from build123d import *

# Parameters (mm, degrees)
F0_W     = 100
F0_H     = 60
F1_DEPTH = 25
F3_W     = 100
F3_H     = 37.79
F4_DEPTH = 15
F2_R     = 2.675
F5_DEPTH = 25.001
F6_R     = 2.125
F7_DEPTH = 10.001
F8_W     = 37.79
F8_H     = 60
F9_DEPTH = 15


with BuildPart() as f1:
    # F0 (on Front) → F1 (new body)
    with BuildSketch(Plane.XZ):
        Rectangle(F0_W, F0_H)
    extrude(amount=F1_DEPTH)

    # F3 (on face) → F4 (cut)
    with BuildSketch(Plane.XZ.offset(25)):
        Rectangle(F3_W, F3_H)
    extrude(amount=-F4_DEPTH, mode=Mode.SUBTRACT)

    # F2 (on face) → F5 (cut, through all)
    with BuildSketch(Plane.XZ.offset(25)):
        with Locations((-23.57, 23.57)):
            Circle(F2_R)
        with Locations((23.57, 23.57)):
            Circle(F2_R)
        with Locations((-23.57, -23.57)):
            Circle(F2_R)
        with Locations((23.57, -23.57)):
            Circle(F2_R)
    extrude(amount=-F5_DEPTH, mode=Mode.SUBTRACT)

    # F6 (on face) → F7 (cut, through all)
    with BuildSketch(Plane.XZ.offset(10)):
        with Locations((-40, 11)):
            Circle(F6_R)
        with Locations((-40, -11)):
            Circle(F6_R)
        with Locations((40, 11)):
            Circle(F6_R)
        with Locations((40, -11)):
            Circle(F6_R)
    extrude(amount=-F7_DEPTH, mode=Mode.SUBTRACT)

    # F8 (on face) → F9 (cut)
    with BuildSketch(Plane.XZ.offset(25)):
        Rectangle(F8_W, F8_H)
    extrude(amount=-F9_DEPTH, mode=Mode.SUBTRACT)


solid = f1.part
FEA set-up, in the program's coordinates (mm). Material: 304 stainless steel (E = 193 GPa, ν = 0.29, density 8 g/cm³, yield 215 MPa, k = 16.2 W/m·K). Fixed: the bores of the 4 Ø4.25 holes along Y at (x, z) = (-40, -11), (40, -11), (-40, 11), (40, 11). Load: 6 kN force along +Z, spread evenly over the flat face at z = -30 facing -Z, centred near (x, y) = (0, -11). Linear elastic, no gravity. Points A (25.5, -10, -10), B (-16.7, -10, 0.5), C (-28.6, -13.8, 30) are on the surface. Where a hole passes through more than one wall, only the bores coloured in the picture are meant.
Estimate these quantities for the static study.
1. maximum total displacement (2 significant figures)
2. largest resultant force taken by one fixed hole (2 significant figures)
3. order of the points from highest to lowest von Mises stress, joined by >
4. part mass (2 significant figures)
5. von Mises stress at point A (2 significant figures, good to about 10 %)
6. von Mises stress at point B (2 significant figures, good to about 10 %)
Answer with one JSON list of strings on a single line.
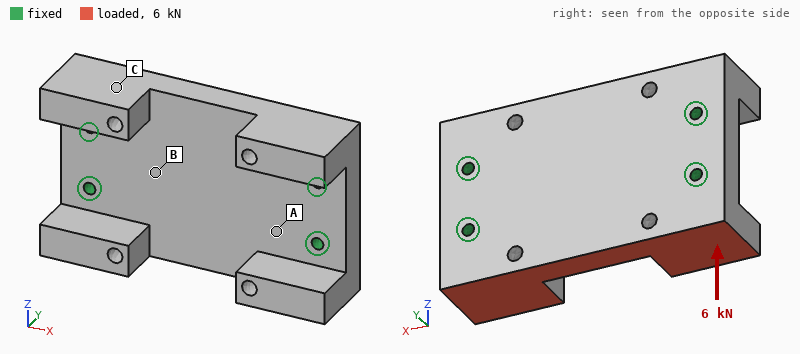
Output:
["15 µm", "2.1 kN", "A > B > C", "620 g", "18 MPa", "9.5 MPa"]
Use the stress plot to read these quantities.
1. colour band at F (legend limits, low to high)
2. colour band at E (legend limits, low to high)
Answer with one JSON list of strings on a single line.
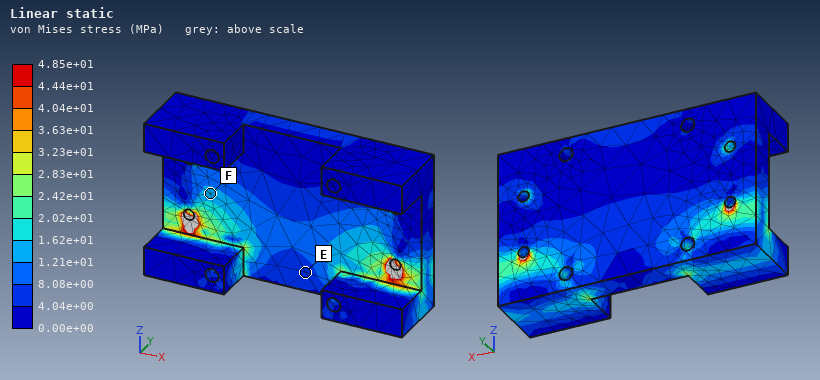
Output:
["1.21e+01 to 1.62e+01 MPa", "4.04e+00 to 8.08e+00 MPa"]
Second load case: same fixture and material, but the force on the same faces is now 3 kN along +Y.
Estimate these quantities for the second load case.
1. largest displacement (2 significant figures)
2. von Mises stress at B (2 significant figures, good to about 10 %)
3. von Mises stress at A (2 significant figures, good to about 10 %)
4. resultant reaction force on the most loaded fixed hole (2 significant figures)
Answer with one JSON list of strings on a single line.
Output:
["20 µm", "13 MPa", "20 MPa", "2.0 kN"]
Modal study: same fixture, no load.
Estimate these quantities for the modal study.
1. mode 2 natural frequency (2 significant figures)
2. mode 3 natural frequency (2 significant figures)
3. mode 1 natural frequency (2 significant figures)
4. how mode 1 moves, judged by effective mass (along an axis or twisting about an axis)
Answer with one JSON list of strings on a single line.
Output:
["5900 Hz", "8700 Hz", "5600 Hz", "along Y"]
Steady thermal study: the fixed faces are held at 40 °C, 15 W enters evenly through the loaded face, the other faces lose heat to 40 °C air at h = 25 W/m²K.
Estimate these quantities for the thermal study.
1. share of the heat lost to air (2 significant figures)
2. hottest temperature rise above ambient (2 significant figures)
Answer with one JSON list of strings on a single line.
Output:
["25 %", "25 K"]
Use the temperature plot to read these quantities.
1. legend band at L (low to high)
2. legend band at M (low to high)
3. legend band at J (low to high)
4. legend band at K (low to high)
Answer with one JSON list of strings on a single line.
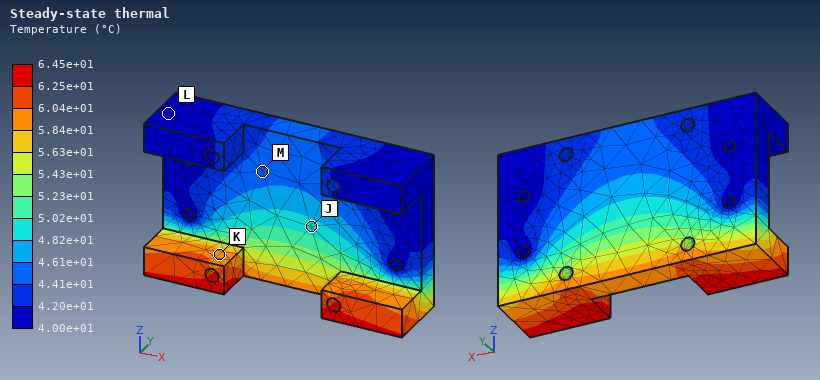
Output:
["4.00e+01 to 4.20e+01 °C", "4.41e+01 to 4.61e+01 °C", "4.82e+01 to 5.02e+01 °C", "5.84e+01 to 6.04e+01 °C"]
